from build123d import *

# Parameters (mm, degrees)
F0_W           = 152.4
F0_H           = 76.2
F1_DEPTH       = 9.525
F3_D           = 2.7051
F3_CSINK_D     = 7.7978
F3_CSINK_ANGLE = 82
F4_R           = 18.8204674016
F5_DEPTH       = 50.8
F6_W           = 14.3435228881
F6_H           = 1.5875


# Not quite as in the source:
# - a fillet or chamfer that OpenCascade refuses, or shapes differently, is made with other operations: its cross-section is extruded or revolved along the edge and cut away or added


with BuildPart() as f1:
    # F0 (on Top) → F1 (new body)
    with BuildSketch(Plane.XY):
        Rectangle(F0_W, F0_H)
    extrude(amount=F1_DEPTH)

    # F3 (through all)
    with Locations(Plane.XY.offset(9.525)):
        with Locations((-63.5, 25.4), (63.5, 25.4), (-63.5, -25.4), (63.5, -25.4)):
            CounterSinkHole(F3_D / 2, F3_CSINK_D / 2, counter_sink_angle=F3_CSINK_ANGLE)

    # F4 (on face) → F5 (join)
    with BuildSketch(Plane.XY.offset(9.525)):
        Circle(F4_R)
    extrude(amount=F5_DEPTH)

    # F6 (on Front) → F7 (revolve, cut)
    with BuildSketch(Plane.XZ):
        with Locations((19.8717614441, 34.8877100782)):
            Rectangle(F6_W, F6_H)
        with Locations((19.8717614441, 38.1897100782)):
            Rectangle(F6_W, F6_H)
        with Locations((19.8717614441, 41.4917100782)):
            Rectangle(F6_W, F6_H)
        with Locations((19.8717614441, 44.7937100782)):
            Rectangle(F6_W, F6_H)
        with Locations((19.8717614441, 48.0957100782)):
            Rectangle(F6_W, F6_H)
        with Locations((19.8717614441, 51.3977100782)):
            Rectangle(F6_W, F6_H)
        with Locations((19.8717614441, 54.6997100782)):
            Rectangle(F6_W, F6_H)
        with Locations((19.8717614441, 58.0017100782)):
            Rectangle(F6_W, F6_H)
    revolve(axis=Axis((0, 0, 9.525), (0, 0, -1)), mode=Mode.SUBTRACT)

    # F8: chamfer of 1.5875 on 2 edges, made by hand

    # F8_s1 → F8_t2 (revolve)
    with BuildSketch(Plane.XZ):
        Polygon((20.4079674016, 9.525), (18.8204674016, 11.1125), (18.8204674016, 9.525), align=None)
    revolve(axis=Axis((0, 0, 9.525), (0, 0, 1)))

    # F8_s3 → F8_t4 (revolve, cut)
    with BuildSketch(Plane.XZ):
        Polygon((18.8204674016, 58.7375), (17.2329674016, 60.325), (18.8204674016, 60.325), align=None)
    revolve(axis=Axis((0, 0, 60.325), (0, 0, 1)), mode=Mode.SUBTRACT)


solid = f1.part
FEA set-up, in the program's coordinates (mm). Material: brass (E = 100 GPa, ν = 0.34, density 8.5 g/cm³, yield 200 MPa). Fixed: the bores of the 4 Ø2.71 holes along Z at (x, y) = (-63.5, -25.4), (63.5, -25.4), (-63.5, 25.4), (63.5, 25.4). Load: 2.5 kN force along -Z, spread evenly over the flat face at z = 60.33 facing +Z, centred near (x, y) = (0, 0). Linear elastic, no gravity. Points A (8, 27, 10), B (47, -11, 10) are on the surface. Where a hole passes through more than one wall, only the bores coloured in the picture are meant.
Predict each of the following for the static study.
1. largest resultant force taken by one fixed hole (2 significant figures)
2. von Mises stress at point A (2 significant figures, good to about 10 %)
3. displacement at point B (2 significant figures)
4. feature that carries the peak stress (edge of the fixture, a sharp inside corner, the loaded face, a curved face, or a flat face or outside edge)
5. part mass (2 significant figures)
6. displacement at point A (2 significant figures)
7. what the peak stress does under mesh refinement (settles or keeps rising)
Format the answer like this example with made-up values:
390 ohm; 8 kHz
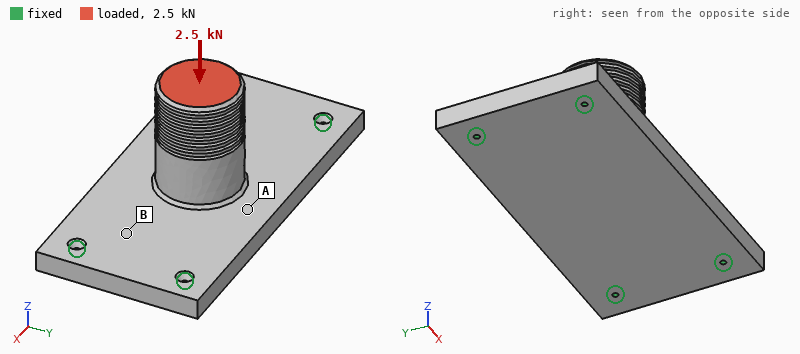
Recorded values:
930 N; 18 MPa; 23 µm; edge of the fixture; 1.4 kg; 56 µm; keeps rising
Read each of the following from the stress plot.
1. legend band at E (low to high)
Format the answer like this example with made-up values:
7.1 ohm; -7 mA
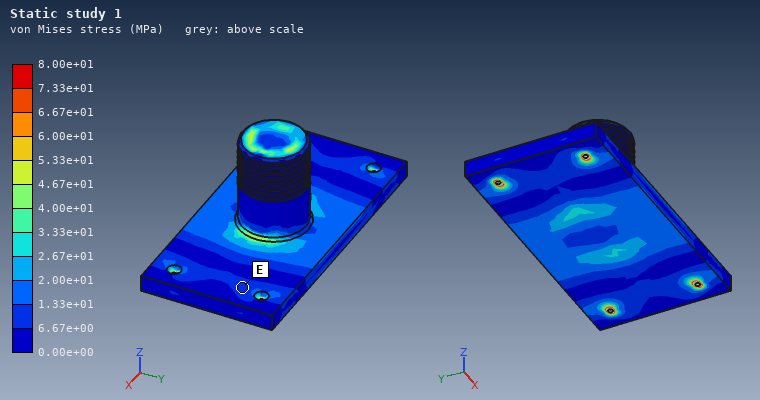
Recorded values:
6.67e+00 to 1.33e+01 MPa
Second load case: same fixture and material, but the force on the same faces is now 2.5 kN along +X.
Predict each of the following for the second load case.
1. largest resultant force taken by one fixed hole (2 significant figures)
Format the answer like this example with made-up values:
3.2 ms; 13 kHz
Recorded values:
930 N
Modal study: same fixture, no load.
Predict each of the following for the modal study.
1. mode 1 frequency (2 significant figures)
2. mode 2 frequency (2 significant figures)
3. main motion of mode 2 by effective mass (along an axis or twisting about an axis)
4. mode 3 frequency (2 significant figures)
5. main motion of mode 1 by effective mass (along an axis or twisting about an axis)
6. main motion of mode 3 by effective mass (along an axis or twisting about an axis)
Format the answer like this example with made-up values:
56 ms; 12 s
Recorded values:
1200 Hz; 1300 Hz; along Y; 2100 Hz; along Z; along X
